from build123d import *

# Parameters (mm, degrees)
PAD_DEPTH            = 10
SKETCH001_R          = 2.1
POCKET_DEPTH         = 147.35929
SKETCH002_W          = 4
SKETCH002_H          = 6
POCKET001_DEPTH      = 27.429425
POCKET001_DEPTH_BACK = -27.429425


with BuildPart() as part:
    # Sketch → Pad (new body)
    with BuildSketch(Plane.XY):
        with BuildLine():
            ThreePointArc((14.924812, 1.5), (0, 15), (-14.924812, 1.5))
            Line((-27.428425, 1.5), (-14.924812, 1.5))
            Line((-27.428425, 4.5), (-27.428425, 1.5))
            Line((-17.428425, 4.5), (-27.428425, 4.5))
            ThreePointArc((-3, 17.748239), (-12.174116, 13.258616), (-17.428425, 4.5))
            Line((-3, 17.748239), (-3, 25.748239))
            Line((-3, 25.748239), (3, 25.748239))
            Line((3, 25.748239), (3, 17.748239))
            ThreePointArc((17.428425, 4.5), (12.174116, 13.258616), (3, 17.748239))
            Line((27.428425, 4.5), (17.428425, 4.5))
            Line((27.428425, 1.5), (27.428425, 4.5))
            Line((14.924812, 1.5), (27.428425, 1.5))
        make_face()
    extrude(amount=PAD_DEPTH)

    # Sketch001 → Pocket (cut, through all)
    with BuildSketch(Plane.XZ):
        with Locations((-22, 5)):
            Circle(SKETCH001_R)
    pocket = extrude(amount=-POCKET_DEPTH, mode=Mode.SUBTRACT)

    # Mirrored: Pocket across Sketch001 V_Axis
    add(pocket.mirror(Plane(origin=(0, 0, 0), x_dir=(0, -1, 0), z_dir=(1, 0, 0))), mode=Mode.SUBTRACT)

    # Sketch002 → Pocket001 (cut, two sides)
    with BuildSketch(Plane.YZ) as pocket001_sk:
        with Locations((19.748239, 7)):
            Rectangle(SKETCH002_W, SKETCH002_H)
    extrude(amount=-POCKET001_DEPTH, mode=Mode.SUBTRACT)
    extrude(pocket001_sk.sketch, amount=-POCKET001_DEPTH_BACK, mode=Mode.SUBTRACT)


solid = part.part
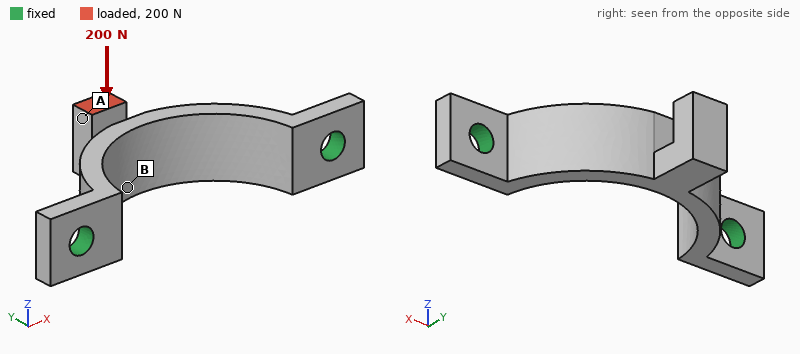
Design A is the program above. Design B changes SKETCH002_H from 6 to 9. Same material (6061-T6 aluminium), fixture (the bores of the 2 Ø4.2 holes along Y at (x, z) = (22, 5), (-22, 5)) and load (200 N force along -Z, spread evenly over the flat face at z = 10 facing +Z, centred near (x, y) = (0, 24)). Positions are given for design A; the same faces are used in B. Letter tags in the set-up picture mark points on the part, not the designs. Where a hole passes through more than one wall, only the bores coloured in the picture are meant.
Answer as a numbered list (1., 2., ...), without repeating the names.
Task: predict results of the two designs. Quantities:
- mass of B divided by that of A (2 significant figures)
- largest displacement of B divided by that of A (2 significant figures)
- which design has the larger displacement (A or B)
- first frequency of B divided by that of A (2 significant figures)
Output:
1. 0.98
2. 1.4
3. B
4. 0.97
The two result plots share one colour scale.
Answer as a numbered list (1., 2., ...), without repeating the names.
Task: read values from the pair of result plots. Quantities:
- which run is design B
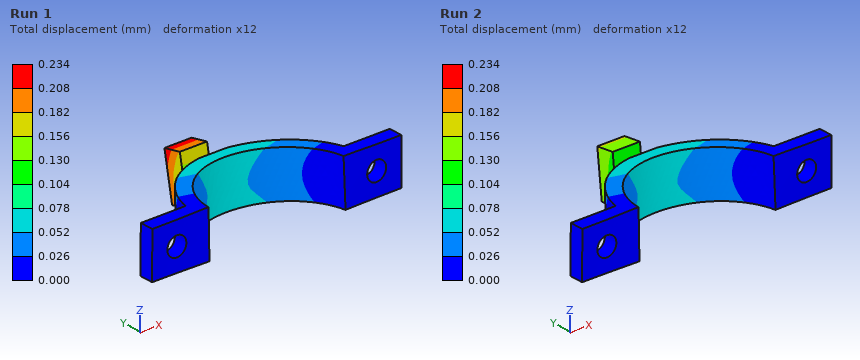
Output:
1. Run 1
